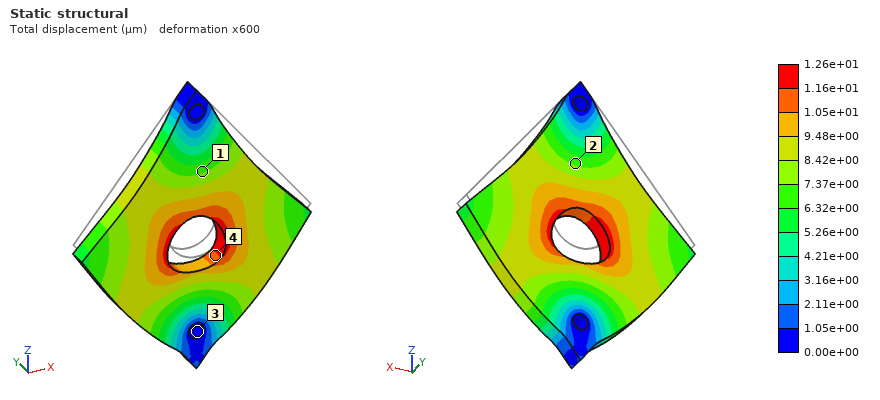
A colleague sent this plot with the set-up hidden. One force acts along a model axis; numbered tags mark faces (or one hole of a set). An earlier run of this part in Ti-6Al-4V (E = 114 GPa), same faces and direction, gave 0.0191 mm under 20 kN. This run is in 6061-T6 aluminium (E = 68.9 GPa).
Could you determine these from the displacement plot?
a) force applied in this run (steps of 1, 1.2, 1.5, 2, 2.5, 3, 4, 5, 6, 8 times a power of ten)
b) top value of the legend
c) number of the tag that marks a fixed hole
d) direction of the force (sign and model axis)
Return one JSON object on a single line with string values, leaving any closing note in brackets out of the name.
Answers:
{"force applied in this run": "8 kN", "top value of the legend": "1.26e+01 µm", "number of the tag that marks a fixed hole": "3", "direction of the force": "-Z"}
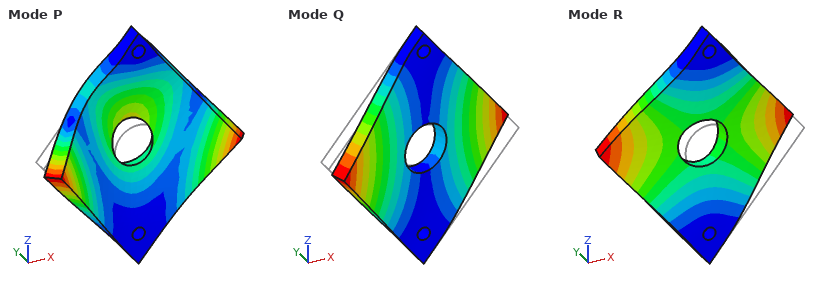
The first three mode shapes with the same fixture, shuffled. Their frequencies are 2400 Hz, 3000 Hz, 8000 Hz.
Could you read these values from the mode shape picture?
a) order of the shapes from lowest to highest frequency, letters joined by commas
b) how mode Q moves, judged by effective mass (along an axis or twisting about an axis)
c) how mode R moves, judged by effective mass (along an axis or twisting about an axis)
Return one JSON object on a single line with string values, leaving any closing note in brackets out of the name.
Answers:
{"order of the shapes from lowest to highest frequency, letters joined by commas": "Q, R, P", "how mode Q moves, judged by effective mass": "twisting about Z", "how mode R moves, judged by effective mass": "along Y"}
